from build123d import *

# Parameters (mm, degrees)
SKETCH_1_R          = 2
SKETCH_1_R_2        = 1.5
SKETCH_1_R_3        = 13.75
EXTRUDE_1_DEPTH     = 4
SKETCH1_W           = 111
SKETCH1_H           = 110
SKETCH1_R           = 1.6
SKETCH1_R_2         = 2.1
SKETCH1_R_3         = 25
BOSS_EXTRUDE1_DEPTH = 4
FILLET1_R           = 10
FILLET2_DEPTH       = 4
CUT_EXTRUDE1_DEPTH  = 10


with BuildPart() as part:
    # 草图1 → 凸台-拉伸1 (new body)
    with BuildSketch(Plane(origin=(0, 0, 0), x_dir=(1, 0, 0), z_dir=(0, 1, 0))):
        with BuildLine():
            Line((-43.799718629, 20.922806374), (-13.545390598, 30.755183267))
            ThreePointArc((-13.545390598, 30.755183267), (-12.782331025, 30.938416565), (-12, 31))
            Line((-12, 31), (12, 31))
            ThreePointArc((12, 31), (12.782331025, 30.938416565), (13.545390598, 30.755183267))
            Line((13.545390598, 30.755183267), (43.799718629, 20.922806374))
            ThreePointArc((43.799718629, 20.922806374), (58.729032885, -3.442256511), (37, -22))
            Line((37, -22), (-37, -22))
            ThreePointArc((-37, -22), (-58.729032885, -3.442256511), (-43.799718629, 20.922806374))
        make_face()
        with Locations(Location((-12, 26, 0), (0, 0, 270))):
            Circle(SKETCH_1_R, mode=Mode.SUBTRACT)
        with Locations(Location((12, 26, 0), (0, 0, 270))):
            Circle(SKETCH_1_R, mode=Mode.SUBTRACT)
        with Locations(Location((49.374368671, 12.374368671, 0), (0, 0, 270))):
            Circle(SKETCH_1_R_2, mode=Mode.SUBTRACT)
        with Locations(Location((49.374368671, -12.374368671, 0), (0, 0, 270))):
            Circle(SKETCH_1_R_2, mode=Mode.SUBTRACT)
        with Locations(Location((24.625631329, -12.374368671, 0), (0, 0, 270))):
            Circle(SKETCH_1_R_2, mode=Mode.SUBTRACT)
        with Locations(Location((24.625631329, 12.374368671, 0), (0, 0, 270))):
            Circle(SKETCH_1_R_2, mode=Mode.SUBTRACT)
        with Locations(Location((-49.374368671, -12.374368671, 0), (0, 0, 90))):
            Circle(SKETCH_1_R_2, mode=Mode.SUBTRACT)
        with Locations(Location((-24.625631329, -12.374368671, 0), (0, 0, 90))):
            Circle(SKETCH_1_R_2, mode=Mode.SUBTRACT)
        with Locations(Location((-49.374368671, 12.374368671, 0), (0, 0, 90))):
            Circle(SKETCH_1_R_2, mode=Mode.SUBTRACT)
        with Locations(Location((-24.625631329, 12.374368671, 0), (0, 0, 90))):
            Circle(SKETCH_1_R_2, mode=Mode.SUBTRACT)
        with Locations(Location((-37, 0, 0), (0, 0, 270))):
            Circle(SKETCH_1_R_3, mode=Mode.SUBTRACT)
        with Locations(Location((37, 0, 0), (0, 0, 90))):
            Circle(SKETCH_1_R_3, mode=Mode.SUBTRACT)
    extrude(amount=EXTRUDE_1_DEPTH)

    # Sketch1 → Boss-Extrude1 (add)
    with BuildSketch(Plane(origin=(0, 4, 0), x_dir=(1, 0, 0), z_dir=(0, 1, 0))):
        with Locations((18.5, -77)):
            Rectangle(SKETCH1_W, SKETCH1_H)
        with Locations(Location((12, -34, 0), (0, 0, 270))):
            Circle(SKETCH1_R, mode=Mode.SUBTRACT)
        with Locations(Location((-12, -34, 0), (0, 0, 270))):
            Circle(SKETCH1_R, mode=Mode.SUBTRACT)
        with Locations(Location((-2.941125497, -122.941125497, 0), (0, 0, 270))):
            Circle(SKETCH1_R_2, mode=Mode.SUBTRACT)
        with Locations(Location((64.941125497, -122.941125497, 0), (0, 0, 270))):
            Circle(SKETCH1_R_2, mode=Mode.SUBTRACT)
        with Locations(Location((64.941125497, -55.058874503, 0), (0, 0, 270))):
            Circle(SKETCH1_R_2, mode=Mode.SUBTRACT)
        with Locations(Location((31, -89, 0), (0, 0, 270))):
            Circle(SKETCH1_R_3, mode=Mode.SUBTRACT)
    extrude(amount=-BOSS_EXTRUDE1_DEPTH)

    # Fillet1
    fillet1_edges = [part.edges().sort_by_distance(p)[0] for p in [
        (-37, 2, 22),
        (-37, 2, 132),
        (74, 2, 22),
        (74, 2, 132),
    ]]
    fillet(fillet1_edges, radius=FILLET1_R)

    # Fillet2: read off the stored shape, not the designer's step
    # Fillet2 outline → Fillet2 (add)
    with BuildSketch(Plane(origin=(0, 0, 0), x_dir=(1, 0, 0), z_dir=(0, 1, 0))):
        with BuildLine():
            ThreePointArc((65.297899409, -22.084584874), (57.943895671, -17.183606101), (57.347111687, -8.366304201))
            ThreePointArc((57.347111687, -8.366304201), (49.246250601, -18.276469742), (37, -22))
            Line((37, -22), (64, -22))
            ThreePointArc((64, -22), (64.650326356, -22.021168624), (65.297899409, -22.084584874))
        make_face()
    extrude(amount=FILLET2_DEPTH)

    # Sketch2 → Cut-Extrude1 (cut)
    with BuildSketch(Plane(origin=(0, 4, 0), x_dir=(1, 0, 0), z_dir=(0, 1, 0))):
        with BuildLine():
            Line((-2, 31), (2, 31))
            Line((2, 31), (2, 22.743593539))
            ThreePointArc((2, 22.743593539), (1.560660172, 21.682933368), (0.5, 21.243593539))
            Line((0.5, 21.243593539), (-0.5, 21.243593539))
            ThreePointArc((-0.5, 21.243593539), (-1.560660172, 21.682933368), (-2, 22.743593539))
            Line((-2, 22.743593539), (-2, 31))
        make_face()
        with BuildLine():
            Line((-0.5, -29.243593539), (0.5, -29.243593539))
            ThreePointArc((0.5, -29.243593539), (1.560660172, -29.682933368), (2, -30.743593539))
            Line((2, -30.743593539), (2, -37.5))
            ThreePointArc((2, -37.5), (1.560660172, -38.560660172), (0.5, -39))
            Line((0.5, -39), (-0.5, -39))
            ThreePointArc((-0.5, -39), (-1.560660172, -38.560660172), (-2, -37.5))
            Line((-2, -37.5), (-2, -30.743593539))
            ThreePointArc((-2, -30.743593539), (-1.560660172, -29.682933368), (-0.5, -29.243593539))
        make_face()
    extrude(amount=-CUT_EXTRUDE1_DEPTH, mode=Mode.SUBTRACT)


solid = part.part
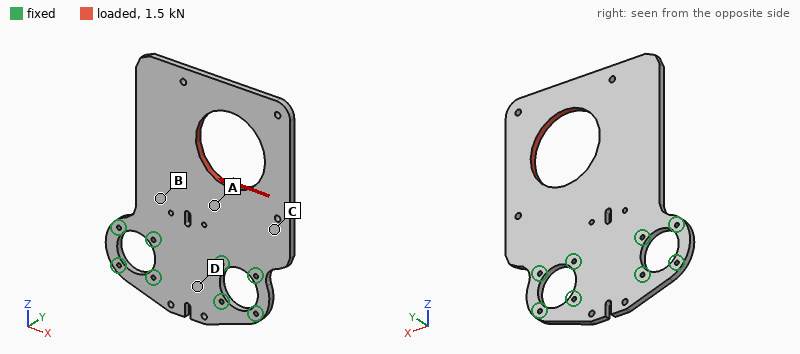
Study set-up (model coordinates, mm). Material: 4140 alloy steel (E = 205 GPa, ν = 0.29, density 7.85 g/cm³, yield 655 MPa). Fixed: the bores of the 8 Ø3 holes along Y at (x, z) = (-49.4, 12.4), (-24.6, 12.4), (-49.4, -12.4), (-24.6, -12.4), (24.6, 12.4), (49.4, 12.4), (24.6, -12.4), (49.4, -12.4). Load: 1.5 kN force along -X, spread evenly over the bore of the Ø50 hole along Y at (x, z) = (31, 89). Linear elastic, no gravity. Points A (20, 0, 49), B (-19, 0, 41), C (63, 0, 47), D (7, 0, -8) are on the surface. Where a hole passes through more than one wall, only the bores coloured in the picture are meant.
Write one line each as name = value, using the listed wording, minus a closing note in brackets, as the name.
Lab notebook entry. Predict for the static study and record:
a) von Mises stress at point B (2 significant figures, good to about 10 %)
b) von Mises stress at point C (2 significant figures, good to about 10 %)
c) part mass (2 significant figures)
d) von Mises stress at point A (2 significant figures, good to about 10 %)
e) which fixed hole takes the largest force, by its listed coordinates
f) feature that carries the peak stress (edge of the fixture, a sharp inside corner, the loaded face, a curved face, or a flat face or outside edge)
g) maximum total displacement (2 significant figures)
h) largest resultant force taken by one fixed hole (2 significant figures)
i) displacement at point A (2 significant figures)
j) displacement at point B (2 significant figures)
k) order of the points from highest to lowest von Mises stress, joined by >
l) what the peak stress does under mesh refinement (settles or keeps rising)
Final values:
von Mises stress at point B = 9.1 MPa
von Mises stress at point C = 4.9 MPa
part mass = 440 g
von Mises stress at point A = 14 MPa
which fixed hole takes the largest force, by its listed coordinates = (49.4, 12.4)
feature that carries the peak stress = edge of the fixture
maximum total displacement = 19 µm
largest resultant force taken by one fixed hole = 1.2 kN
displacement at point A = 4.2 µm
displacement at point B = 3.1 µm
order of the points from highest to lowest von Mises stress, joined by > = A > B > C > D
what the peak stress does under mesh refinement = keeps rising
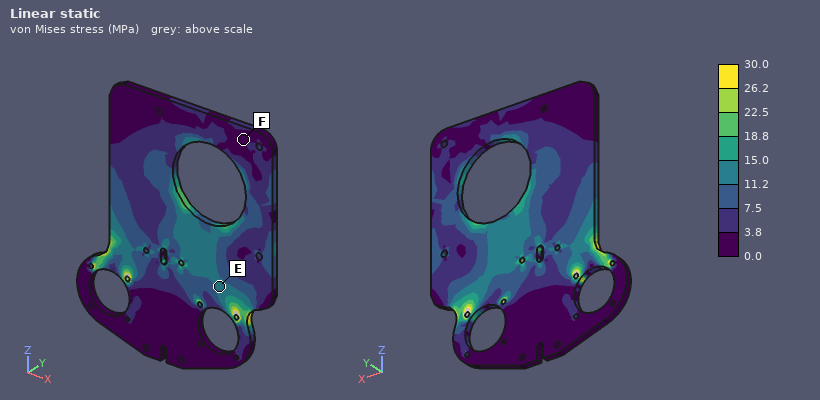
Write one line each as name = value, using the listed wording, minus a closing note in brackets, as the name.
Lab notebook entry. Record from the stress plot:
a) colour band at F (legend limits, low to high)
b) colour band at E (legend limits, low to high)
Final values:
colour band at F = 0.0 to 3.8 MPa
colour band at E = 11.2 to 15.0 MPa
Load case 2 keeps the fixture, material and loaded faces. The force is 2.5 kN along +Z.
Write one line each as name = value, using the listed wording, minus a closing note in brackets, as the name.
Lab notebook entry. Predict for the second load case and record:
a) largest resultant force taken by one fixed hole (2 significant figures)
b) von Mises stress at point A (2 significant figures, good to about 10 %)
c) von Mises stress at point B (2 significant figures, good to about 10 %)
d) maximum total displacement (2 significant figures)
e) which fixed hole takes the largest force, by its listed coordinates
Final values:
largest resultant force taken by one fixed hole = 1.2 kN
von Mises stress at point A = 8.7 MPa
von Mises stress at point B = 3.4 MPa
maximum total displacement = 10 µm
which fixed hole takes the largest force, by its listed coordinates = (49.4, 12.4)
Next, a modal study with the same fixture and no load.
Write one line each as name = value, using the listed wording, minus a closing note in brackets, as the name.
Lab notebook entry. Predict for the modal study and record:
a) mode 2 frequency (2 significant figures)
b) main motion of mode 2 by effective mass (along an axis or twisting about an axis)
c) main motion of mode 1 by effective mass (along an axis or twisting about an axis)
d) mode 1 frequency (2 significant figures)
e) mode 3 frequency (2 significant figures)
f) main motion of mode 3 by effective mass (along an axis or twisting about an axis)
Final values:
mode 2 frequency = 540 Hz
main motion of mode 2 by effective mass = twisting about Z
main motion of mode 1 by effective mass = along Y
mode 1 frequency = 230 Hz
mode 3 frequency = 1200 Hz
main motion of mode 3 by effective mass = along Y
